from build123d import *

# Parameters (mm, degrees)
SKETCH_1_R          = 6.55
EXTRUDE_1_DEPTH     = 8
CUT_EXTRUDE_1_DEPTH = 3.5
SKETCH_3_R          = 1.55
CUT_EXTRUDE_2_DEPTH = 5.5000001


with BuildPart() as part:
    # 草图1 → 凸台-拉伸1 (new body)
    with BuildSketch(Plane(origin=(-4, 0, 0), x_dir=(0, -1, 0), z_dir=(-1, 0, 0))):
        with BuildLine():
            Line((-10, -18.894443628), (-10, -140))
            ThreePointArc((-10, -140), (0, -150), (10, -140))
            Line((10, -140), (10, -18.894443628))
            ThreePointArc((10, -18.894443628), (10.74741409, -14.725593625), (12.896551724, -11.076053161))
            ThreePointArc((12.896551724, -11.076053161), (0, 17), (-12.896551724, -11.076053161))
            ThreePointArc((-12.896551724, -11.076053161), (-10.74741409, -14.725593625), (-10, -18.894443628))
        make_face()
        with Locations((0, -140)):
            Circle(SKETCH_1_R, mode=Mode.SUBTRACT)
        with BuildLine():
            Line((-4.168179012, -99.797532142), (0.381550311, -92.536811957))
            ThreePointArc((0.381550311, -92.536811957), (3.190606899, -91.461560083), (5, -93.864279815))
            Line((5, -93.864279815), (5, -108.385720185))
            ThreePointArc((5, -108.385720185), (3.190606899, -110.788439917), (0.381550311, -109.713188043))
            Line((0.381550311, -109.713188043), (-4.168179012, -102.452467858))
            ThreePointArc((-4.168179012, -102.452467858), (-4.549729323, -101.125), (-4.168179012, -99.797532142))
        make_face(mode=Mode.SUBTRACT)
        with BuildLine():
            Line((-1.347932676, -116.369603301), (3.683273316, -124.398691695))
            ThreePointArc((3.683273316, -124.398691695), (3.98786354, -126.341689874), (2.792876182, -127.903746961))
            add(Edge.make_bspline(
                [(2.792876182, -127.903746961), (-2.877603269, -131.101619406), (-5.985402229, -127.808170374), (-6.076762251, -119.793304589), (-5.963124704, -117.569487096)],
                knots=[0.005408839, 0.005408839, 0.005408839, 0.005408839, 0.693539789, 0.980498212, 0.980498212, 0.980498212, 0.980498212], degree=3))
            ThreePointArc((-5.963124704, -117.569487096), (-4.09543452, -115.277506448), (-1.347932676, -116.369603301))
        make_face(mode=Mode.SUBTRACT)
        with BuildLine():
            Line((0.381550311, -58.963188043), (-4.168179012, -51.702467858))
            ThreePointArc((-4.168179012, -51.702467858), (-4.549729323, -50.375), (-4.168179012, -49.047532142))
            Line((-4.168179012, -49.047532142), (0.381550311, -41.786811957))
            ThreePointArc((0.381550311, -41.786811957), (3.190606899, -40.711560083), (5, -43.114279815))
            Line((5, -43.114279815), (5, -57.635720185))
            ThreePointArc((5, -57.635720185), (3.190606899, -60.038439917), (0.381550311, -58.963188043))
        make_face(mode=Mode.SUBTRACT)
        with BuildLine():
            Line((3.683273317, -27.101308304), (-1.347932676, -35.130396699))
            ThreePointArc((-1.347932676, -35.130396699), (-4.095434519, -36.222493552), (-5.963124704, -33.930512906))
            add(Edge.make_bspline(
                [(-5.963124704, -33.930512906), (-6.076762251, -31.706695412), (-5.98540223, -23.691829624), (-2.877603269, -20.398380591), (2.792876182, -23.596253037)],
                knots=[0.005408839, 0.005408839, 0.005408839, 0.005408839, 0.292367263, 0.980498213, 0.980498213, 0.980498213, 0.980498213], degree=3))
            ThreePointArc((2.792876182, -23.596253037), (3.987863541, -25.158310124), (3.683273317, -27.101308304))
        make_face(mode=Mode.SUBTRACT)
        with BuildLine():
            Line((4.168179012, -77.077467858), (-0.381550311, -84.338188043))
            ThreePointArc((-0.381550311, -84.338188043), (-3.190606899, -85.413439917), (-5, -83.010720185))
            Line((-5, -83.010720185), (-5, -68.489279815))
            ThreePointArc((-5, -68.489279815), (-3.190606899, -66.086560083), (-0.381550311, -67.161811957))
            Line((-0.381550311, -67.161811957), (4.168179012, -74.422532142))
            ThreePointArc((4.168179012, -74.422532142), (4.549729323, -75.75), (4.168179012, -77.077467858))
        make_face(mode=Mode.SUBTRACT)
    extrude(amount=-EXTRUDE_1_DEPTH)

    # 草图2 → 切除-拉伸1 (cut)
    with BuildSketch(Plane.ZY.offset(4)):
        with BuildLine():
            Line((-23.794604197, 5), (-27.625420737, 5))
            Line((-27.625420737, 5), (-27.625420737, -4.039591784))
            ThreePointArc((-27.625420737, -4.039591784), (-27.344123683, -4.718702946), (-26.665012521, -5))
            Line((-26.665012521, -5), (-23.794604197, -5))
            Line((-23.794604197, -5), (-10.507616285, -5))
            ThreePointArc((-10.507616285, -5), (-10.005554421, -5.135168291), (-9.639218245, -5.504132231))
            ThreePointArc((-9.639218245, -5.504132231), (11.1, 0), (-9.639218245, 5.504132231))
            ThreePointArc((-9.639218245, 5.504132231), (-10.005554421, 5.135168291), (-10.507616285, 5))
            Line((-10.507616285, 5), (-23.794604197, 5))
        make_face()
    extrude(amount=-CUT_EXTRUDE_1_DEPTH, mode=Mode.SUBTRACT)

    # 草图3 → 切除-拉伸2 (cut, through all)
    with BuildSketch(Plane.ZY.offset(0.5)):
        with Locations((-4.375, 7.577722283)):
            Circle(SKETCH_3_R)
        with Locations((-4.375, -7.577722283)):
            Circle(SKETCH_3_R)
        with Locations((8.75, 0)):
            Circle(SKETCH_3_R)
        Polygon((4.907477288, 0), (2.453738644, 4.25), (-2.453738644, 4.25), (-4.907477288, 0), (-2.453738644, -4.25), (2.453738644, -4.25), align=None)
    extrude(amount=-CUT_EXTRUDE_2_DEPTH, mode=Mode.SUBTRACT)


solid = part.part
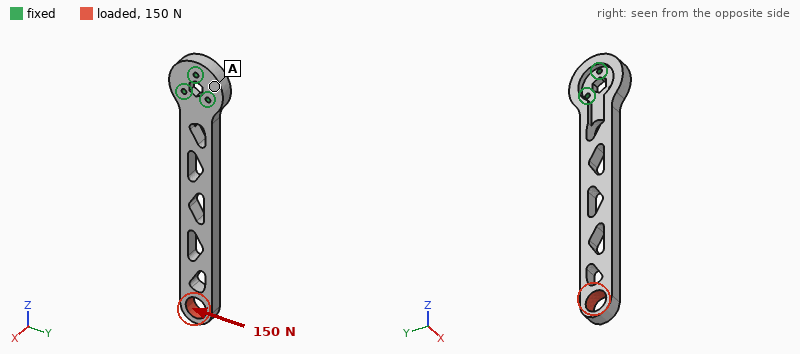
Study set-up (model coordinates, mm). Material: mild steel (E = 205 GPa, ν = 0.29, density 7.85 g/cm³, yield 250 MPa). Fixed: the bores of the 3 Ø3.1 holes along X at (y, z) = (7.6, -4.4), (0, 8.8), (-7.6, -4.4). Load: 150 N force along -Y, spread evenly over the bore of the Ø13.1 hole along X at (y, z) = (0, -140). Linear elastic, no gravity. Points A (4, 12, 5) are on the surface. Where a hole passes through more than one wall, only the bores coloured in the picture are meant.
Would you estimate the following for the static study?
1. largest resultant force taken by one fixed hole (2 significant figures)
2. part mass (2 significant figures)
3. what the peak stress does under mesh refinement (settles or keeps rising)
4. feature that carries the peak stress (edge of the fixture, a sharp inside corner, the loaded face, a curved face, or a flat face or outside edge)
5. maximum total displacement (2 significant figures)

1.1 kN
160 g
keeps rising
edge of the fixture
0.14 mm
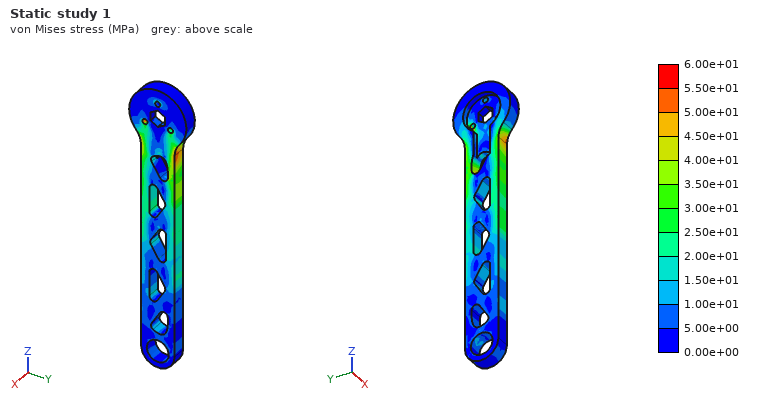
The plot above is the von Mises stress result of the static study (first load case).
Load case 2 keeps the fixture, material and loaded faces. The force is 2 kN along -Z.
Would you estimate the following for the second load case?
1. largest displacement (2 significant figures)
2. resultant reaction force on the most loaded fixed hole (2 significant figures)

50 µm
980 N
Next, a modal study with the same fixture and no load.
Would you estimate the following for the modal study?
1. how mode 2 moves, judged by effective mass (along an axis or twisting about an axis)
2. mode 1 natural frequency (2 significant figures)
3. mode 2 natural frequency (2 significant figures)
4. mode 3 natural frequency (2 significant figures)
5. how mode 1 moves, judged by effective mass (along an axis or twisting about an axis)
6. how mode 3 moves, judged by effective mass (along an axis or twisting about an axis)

along Y
300 Hz
910 Hz
1800 Hz
along X
along X
